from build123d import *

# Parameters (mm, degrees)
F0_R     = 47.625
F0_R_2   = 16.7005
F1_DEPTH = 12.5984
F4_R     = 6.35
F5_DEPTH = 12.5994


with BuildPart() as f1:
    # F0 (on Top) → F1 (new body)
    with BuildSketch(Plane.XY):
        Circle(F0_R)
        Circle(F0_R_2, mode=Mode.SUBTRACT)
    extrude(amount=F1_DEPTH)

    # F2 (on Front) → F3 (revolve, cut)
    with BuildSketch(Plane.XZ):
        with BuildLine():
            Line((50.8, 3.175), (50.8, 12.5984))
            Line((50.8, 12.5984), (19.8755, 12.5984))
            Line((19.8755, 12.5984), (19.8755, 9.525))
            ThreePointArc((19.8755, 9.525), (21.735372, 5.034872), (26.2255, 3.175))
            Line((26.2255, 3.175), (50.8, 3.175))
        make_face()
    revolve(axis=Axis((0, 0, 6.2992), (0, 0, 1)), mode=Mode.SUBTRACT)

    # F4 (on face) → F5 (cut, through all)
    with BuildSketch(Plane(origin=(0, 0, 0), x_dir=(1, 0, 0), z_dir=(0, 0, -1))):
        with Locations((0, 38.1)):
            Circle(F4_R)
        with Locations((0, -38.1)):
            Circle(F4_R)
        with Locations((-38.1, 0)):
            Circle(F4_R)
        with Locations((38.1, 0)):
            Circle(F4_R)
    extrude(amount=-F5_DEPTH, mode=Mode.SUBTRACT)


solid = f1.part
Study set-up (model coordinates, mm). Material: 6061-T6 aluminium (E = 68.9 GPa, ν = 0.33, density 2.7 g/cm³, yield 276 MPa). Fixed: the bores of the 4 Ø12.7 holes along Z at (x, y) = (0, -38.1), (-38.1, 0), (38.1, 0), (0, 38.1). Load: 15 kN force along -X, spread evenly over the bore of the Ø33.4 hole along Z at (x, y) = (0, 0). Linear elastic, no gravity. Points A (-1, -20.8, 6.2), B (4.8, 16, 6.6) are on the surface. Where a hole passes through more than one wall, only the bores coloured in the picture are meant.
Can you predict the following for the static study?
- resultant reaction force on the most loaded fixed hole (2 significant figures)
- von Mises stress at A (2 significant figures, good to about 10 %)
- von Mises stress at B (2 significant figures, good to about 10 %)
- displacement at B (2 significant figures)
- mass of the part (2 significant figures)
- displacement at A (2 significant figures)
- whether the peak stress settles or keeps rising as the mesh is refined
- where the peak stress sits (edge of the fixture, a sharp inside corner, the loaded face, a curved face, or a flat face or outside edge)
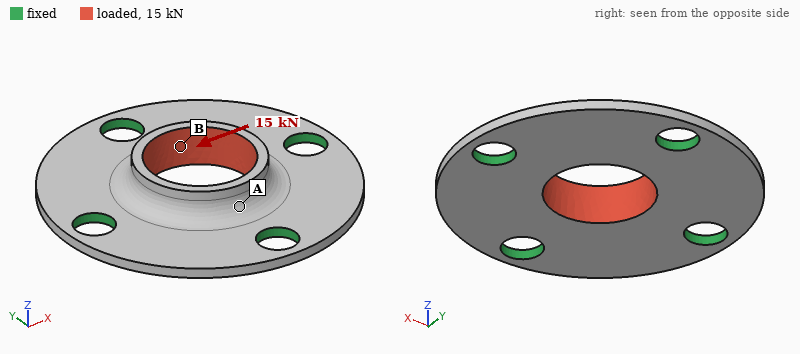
4.7 kN
25 MPa
56 MPa
27 µm
62 g
21 µm
keeps rising
edge of the fixture
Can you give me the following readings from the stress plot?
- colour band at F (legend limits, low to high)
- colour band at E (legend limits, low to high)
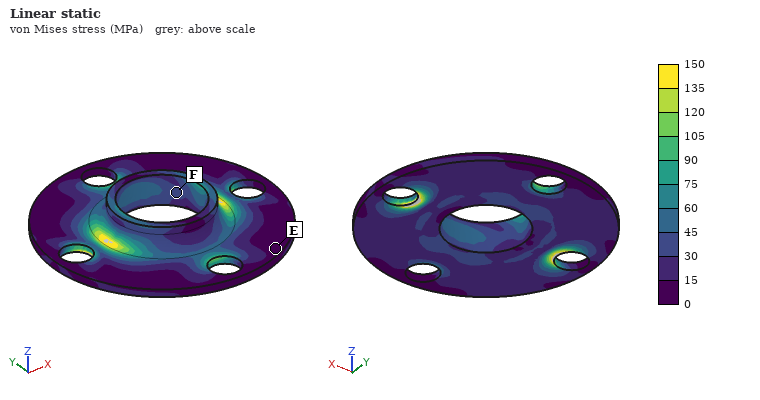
30 to 45 MPa
0 to 15 MPa
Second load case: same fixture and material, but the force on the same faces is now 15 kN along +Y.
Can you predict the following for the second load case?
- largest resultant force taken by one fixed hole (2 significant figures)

4.7 kN
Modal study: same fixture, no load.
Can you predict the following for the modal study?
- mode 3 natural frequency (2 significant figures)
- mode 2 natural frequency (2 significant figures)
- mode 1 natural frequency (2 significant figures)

6500 Hz
6500 Hz
6400 Hz
